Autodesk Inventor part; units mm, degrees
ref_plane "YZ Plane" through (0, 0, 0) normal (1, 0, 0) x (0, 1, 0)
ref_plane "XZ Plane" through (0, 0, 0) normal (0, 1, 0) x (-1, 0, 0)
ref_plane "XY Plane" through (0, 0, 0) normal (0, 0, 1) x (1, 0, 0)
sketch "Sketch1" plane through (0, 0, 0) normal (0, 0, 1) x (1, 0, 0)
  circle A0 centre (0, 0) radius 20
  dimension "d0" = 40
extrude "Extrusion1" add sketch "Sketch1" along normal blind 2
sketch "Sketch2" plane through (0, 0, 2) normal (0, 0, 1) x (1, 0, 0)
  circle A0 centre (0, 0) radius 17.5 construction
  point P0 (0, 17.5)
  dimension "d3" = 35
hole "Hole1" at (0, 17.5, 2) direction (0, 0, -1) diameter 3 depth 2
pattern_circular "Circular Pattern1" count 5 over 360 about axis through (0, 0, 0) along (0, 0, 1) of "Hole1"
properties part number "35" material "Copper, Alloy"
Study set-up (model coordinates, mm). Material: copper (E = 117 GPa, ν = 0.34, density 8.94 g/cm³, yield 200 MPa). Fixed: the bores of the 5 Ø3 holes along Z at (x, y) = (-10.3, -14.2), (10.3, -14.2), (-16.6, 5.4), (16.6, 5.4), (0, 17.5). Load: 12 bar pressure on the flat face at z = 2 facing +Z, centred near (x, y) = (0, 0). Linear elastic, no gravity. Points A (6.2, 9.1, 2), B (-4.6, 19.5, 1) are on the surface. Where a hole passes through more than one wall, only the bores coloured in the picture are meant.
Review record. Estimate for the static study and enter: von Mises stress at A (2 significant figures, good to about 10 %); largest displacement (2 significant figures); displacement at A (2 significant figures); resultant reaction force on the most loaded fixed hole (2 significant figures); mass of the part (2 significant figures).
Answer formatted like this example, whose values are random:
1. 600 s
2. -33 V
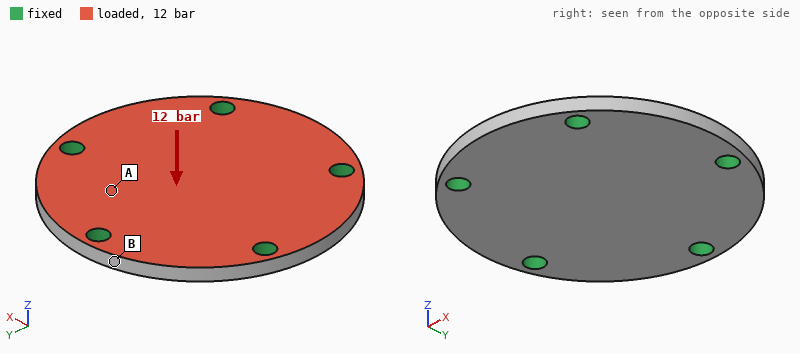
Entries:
1. 37 MPa
2. 25 µm
3. 13 µm
4. 290 N
5. 22 g
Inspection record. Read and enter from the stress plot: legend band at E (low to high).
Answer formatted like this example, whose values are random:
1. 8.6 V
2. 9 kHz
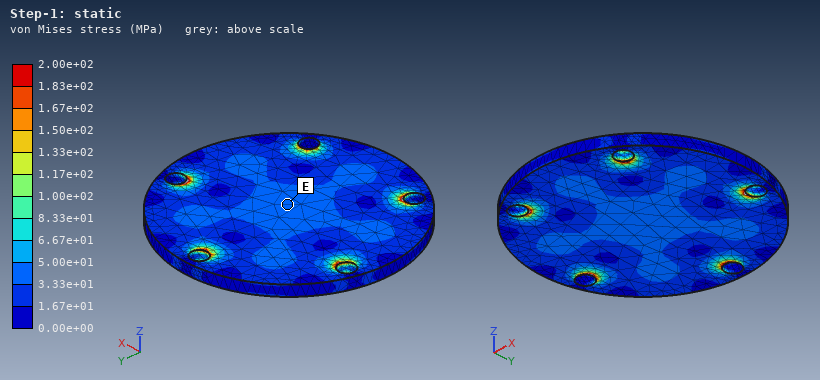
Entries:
1. 3.33e+01 to 5.00e+01 MPa
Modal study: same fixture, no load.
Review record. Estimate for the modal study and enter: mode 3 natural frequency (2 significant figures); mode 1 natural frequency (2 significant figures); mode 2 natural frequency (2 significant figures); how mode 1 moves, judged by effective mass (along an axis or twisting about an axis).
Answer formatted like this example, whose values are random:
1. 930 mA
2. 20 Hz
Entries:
1. 17 kHz
2. 10 kHz
3. 17 kHz
4. along Z
